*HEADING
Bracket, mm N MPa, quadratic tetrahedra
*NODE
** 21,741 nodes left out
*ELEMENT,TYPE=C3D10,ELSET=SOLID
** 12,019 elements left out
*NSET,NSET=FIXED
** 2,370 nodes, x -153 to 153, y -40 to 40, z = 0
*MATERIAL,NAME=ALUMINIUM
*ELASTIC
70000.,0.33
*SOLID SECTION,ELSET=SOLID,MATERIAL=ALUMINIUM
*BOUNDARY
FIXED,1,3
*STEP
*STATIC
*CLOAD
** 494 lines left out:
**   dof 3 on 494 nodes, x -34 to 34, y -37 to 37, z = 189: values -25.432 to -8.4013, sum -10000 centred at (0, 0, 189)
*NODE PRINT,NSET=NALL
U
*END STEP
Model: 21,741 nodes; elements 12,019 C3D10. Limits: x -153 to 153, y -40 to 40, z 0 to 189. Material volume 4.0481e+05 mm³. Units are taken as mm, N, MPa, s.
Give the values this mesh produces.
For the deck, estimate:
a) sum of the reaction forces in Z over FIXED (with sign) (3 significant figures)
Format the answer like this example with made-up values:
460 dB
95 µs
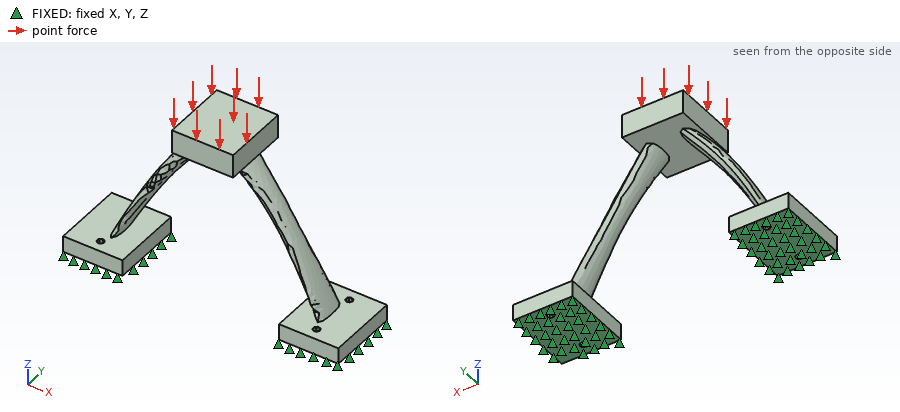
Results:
10000 N
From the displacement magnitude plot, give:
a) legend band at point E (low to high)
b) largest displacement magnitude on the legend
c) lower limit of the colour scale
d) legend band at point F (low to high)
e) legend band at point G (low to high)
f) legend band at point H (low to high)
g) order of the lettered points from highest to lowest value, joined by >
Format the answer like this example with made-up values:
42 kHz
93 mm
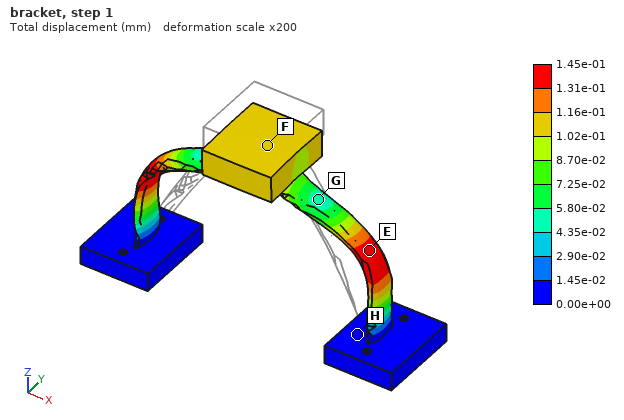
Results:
1.31e-01 to 1.45e-01 mm
1.45e-01 mm
0.00e+00 mm
1.02e-01 to 1.16e-01 mm
4.35e-02 to 5.80e-02 mm
0.00e+00 to 1.45e-02 mm
E > F > G > H
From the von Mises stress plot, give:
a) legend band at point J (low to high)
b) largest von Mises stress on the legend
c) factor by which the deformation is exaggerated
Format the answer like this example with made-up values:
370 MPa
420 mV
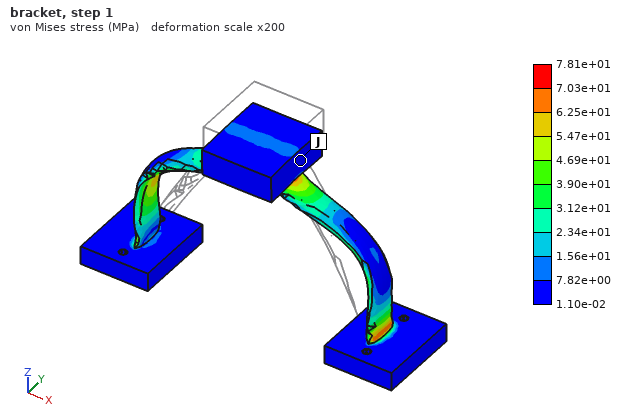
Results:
1.10e-02 to 7.82e+00 MPa
7.81e+01 MPa
200
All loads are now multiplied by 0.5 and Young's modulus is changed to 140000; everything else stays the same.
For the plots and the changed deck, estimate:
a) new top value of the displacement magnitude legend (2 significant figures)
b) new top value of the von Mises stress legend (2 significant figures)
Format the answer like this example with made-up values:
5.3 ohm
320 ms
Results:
0.036 mm
39 MPa
